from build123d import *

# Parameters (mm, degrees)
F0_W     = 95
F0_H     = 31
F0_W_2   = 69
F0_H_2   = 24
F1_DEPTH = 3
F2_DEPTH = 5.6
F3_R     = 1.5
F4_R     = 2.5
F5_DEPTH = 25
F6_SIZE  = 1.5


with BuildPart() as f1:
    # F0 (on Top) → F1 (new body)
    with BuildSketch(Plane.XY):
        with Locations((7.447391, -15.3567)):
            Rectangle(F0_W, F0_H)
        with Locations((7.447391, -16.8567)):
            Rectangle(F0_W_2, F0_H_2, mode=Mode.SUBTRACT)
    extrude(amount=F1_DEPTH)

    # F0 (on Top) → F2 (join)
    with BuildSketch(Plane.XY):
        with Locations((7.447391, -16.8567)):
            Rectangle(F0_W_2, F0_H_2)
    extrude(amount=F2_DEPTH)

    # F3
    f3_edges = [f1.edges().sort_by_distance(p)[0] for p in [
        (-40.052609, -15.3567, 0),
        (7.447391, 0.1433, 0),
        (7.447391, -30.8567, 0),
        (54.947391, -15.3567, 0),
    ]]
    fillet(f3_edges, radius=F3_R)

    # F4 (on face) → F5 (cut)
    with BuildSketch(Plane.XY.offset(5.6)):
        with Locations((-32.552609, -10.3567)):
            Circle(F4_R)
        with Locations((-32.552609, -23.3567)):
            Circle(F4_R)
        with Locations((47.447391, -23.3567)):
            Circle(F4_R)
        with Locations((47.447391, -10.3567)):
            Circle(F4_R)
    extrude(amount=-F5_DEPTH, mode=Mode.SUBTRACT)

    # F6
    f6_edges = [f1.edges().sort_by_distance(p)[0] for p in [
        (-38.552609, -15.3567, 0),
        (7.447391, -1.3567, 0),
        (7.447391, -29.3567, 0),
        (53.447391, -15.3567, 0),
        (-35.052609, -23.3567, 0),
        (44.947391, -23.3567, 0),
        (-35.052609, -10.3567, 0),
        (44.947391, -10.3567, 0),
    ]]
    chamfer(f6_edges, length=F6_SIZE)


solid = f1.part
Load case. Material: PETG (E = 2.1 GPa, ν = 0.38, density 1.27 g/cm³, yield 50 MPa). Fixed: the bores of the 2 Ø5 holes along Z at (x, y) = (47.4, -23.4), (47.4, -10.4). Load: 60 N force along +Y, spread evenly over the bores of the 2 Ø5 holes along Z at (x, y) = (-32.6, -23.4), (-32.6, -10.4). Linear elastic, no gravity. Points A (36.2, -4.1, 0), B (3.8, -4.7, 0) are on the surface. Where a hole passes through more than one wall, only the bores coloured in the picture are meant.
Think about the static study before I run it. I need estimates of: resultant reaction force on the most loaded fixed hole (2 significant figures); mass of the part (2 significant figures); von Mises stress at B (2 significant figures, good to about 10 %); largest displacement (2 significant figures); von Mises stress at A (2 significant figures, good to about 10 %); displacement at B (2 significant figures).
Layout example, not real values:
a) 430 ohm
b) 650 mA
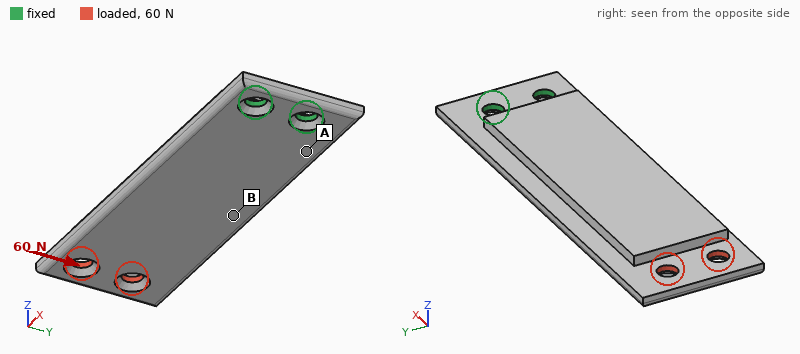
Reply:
a) 300 N
b) 16 g
c) 2.3 MPa
d) 0.94 mm
e) 4.9 MPa
f) 0.38 mm
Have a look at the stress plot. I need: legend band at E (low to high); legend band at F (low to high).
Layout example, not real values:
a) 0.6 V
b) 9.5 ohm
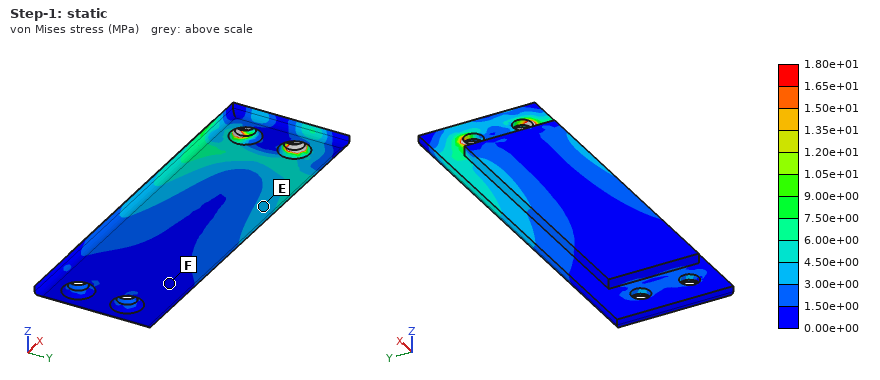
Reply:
a) 3.00e+00 to 4.50e+00 MPa
b) 0.00e+00 to 1.50e+00 MPa
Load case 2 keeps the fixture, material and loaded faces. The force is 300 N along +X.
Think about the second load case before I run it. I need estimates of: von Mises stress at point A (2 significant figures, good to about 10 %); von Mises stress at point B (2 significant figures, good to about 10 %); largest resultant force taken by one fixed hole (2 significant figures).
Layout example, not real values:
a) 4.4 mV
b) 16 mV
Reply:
a) 1.9 MPa
b) 2.4 MPa
c) 150 N
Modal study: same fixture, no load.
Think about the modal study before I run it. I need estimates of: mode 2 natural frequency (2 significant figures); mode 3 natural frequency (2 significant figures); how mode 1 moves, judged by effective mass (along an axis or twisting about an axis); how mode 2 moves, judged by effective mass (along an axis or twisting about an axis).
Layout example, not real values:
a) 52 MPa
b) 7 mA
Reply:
a) 620 Hz
b) 780 Hz
c) along Z
d) along Y
